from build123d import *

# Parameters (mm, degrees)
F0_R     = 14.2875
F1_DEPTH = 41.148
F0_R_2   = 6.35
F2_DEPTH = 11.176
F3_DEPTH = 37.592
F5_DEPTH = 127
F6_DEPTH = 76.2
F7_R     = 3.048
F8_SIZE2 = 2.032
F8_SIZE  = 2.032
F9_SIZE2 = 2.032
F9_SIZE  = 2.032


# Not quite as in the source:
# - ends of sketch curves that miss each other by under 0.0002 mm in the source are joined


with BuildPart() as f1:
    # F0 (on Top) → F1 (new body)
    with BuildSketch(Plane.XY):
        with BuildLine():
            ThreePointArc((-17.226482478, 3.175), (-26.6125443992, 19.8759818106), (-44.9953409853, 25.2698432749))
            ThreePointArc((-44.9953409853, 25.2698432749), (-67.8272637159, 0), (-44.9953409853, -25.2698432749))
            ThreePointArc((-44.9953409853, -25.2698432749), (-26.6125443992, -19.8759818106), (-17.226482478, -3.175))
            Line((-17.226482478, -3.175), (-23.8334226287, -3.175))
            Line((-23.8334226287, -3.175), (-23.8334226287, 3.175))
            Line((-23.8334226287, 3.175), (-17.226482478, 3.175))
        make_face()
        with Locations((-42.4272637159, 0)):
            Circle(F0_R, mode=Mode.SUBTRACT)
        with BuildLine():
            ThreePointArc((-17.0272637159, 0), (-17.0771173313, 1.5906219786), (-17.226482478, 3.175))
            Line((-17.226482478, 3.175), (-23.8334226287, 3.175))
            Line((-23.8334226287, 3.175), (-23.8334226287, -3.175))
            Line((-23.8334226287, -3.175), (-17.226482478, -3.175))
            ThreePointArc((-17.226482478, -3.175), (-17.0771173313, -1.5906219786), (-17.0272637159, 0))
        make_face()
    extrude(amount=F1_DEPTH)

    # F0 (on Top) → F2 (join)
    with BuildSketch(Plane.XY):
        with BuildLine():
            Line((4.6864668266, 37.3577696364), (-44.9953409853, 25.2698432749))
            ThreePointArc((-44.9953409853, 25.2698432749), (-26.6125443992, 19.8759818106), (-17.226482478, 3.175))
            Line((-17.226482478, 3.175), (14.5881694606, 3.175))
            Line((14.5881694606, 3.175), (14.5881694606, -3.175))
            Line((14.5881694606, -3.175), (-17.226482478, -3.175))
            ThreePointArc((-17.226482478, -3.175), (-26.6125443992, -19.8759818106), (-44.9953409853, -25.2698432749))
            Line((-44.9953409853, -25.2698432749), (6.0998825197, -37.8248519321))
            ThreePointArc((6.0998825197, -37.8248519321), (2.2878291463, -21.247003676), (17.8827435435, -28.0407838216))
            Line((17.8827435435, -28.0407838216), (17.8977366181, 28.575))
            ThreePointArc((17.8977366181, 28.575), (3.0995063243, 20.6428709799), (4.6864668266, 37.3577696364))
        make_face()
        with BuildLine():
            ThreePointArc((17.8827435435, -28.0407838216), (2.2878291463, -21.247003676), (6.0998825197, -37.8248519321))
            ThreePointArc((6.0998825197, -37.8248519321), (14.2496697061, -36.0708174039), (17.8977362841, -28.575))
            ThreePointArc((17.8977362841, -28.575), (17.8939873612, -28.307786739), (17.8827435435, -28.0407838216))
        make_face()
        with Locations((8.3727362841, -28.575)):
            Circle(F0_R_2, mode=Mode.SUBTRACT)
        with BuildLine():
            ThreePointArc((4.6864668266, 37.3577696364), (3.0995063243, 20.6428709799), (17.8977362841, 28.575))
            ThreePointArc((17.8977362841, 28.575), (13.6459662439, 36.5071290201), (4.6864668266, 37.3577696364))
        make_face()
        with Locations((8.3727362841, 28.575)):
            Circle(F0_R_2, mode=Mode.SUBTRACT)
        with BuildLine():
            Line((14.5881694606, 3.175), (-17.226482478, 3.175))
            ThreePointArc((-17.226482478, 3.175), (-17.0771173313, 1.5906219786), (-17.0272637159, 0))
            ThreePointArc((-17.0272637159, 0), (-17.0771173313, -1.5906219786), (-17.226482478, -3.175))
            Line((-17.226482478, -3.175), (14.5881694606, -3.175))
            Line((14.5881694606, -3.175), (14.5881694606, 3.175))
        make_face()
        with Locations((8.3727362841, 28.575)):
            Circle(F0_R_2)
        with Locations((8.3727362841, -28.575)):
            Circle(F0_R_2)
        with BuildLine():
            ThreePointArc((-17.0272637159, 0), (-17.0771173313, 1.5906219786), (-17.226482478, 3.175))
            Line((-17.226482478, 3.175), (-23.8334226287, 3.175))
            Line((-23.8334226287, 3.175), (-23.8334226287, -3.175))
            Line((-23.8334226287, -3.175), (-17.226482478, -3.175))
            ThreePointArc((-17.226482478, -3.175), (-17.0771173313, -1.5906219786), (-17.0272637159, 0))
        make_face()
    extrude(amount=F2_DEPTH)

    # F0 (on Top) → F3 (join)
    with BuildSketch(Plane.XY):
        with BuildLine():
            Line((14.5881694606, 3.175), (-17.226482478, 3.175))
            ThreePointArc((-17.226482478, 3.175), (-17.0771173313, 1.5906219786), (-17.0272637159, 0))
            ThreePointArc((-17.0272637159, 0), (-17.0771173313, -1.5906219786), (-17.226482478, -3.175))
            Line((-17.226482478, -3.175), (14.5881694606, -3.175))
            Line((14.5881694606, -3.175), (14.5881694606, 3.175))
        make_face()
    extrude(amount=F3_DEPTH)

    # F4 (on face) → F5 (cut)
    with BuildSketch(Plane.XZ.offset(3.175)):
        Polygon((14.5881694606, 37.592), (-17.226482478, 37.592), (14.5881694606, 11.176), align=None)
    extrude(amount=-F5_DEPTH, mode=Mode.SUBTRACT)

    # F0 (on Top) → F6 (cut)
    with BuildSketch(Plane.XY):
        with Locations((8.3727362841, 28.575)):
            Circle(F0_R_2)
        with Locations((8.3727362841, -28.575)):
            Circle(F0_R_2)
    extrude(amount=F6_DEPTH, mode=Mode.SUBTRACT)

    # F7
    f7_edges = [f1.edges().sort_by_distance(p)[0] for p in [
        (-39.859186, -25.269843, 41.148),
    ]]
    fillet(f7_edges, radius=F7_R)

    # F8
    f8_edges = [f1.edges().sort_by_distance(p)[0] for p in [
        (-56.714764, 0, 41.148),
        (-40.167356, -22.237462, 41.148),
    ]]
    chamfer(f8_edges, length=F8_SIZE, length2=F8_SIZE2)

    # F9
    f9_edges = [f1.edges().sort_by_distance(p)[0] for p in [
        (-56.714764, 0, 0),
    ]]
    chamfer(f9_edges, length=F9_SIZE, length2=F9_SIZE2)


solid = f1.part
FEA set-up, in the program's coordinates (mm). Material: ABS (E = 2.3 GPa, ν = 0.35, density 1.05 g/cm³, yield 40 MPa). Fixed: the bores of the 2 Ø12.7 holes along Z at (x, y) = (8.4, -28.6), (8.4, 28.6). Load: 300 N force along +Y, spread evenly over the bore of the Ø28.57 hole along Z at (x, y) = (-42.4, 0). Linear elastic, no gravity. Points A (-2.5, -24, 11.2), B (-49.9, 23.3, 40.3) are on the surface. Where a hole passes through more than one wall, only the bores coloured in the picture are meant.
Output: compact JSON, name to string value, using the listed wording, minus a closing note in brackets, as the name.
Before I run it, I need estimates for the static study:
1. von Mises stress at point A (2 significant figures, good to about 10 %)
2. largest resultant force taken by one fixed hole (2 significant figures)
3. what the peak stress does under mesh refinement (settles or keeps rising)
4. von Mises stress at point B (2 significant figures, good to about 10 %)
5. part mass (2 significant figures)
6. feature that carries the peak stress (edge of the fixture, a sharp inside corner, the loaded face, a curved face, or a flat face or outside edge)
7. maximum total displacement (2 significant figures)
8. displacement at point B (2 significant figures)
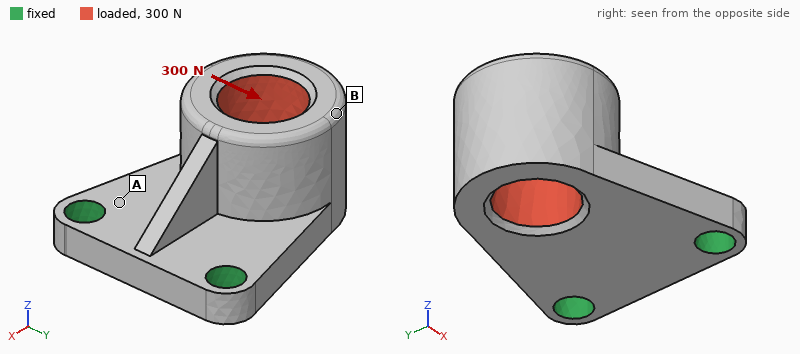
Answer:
{"von Mises stress at point A": "1.2 MPa", "largest resultant force taken by one fixed hole": "300 N", "what the peak stress does under mesh refinement": "keeps rising", "von Mises stress at point B": "0.33 MPa", "part mass": "93 g", "feature that carries the peak stress": "edge of the fixture", "maximum total displacement": "0.14 mm", "displacement at point B": "0.13 mm"}
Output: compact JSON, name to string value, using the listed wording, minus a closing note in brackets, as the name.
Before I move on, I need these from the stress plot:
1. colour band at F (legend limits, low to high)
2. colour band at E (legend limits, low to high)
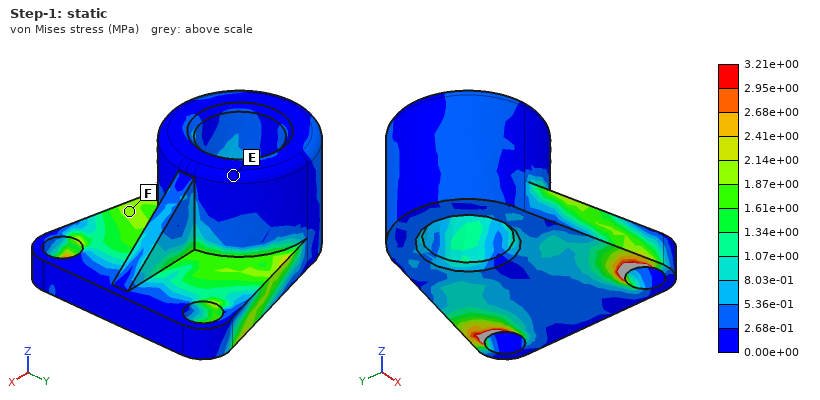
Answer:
{"colour band at F": "1.87e+00 to 2.14e+00 MPa", "colour band at E": "0.00e+00 to 2.68e-01 MPa"}
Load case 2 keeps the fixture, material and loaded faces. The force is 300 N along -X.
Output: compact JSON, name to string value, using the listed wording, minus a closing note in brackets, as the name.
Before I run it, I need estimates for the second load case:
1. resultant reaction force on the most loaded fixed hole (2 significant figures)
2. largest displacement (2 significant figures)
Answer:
{"resultant reaction force on the most loaded fixed hole": "160 N", "largest displacement": "0.35 mm"}
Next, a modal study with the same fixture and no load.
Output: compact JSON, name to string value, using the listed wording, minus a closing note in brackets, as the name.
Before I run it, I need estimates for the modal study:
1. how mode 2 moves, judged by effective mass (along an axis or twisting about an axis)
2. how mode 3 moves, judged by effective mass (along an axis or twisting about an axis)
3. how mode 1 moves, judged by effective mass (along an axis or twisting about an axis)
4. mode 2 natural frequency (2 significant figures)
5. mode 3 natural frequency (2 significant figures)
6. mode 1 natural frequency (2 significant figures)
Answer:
{"how mode 2 moves, judged by effective mass": "along Y", "how mode 3 moves, judged by effective mass": "along Y", "how mode 1 moves, judged by effective mass": "along Z", "mode 2 natural frequency": "1100 Hz", "mode 3 natural frequency": "1800 Hz", "mode 1 natural frequency": "420 Hz"}
